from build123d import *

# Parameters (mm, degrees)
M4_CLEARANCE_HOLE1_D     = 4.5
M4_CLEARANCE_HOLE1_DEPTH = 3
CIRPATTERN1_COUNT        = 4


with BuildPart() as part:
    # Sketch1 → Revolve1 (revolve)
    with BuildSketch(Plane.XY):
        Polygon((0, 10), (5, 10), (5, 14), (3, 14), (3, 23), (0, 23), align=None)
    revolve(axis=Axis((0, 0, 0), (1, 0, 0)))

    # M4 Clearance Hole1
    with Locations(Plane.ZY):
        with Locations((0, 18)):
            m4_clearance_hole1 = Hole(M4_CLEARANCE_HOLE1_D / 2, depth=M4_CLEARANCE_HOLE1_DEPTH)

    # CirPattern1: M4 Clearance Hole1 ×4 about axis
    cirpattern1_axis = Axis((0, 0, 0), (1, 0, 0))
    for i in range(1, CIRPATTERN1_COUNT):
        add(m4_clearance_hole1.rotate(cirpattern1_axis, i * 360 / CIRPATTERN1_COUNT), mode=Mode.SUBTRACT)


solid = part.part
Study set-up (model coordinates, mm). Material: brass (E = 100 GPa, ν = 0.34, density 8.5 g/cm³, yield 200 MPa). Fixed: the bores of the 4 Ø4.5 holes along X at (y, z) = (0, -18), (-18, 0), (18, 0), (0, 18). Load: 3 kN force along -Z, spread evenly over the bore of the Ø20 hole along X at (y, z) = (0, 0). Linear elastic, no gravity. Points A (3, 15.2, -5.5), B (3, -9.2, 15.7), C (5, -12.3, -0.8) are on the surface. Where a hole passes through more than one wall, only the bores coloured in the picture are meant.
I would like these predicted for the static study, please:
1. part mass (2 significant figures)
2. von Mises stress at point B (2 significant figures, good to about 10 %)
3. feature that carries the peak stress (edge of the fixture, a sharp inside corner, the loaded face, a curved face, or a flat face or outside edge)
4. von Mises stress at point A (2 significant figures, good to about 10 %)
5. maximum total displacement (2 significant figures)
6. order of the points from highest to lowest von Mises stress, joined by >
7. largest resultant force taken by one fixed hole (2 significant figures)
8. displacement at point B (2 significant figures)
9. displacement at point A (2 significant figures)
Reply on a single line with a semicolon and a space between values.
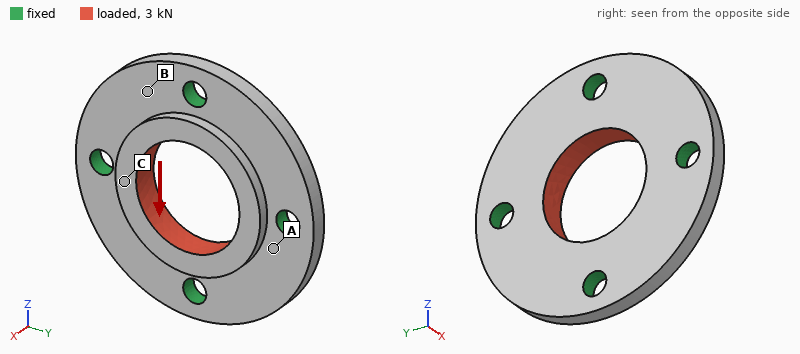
38 g; 9.1 MPa; edge of the fixture; 15 MPa; 3.6 µm; A > B > C; 800 N; 1.9 µm; 1.3 µm
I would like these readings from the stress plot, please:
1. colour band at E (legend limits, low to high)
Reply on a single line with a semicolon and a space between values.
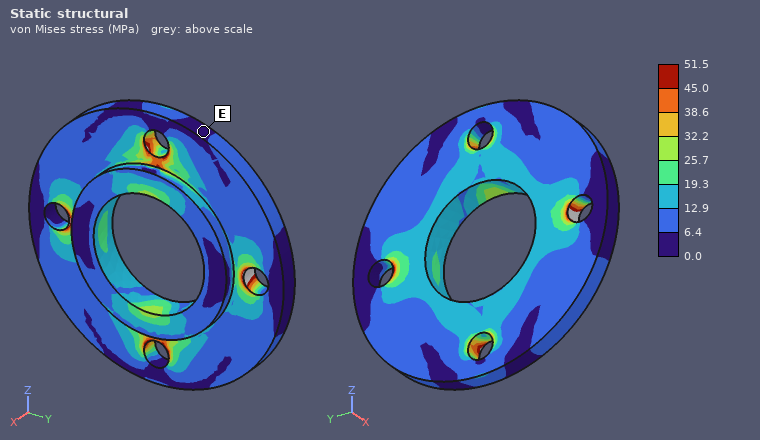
0.0 to 6.4 MPa
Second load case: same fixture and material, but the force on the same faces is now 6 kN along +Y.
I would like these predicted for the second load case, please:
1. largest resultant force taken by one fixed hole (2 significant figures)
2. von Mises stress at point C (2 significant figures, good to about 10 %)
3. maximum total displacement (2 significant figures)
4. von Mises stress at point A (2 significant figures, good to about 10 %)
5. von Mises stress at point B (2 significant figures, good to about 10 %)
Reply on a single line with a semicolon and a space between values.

1.6 kN; 32 MPa; 7.2 µm; 37 MPa; 19 MPa
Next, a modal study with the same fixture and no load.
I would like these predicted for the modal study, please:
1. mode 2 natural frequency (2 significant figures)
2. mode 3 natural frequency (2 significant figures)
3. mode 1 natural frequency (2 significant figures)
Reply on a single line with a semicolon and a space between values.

14 kHz; 14 kHz; 14 kHz
